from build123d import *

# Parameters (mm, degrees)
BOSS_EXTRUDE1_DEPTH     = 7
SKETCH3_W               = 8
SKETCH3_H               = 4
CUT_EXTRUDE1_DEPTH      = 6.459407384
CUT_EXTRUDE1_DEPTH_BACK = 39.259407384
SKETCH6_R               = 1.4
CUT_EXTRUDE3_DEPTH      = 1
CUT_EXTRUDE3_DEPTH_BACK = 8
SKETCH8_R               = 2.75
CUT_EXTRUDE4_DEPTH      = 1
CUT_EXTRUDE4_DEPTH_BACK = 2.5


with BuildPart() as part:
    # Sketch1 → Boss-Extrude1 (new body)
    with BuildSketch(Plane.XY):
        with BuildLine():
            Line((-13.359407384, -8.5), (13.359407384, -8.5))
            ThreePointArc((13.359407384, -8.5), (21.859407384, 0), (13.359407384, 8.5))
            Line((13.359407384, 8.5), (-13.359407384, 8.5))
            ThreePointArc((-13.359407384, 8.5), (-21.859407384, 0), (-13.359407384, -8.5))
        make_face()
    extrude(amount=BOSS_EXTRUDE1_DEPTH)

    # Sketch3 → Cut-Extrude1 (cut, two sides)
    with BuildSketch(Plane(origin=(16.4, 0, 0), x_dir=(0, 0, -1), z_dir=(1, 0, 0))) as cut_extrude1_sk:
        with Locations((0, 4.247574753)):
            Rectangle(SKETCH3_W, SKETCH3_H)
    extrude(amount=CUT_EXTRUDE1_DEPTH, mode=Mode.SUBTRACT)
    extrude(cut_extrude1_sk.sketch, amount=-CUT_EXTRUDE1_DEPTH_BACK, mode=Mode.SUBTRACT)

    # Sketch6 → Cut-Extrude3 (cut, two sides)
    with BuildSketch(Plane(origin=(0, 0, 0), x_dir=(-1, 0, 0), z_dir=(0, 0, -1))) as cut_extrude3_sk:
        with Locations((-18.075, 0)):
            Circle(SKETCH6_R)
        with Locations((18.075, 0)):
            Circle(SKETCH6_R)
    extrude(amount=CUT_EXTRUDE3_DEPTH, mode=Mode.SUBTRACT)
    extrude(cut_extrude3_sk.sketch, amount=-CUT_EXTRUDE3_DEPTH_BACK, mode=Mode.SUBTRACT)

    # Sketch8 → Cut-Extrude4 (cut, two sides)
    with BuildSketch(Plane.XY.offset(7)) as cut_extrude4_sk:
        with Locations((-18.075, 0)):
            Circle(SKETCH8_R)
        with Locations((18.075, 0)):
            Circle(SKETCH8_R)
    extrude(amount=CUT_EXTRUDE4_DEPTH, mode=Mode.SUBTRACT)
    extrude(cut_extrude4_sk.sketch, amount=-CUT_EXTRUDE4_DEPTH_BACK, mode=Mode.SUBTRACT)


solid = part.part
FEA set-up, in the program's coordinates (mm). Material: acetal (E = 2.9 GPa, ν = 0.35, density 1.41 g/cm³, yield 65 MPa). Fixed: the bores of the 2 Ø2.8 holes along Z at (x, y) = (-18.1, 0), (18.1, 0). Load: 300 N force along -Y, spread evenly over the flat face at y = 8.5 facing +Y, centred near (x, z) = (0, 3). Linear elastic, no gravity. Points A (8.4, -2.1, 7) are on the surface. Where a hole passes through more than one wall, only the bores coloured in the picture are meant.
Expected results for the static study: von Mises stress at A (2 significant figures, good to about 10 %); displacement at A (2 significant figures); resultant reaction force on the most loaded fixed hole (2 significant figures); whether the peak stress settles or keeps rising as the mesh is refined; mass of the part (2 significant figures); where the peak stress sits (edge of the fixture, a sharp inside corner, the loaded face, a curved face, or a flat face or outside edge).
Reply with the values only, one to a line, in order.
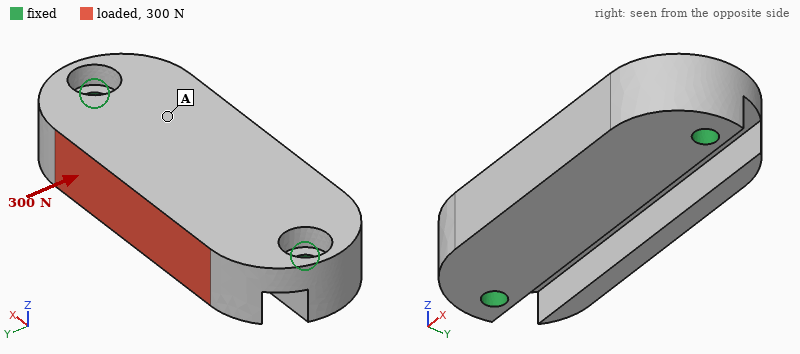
2.6 MPa
0.045 mm
150 N
keeps rising
5.5 g
edge of the fixture
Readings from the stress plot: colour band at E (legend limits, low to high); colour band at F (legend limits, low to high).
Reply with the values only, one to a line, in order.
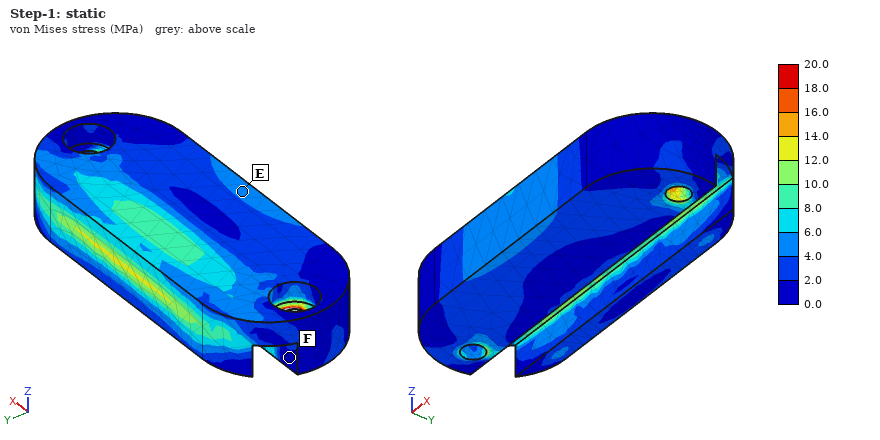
4.0 to 6.0 MPa
0.0 to 2.0 MPa
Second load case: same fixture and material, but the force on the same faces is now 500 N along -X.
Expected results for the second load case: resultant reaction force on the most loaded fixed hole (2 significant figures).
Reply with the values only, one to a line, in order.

280 N
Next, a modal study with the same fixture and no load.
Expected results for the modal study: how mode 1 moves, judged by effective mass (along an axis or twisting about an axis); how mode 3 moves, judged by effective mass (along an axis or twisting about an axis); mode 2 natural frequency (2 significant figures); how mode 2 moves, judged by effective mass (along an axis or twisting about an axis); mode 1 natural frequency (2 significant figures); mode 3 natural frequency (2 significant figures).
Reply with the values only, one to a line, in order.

along Z
along Y
4600 Hz
along Z
3900 Hz
6300 Hz
